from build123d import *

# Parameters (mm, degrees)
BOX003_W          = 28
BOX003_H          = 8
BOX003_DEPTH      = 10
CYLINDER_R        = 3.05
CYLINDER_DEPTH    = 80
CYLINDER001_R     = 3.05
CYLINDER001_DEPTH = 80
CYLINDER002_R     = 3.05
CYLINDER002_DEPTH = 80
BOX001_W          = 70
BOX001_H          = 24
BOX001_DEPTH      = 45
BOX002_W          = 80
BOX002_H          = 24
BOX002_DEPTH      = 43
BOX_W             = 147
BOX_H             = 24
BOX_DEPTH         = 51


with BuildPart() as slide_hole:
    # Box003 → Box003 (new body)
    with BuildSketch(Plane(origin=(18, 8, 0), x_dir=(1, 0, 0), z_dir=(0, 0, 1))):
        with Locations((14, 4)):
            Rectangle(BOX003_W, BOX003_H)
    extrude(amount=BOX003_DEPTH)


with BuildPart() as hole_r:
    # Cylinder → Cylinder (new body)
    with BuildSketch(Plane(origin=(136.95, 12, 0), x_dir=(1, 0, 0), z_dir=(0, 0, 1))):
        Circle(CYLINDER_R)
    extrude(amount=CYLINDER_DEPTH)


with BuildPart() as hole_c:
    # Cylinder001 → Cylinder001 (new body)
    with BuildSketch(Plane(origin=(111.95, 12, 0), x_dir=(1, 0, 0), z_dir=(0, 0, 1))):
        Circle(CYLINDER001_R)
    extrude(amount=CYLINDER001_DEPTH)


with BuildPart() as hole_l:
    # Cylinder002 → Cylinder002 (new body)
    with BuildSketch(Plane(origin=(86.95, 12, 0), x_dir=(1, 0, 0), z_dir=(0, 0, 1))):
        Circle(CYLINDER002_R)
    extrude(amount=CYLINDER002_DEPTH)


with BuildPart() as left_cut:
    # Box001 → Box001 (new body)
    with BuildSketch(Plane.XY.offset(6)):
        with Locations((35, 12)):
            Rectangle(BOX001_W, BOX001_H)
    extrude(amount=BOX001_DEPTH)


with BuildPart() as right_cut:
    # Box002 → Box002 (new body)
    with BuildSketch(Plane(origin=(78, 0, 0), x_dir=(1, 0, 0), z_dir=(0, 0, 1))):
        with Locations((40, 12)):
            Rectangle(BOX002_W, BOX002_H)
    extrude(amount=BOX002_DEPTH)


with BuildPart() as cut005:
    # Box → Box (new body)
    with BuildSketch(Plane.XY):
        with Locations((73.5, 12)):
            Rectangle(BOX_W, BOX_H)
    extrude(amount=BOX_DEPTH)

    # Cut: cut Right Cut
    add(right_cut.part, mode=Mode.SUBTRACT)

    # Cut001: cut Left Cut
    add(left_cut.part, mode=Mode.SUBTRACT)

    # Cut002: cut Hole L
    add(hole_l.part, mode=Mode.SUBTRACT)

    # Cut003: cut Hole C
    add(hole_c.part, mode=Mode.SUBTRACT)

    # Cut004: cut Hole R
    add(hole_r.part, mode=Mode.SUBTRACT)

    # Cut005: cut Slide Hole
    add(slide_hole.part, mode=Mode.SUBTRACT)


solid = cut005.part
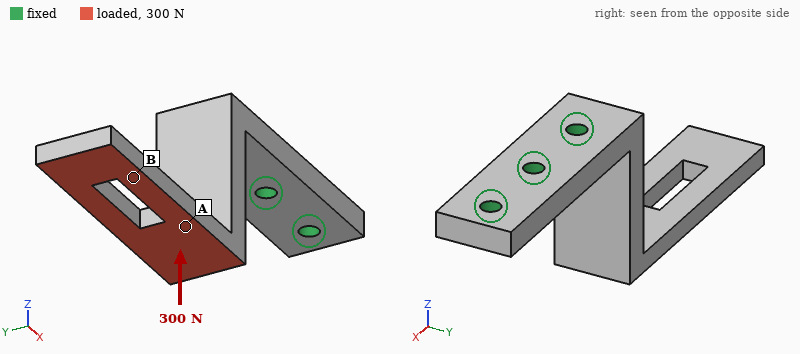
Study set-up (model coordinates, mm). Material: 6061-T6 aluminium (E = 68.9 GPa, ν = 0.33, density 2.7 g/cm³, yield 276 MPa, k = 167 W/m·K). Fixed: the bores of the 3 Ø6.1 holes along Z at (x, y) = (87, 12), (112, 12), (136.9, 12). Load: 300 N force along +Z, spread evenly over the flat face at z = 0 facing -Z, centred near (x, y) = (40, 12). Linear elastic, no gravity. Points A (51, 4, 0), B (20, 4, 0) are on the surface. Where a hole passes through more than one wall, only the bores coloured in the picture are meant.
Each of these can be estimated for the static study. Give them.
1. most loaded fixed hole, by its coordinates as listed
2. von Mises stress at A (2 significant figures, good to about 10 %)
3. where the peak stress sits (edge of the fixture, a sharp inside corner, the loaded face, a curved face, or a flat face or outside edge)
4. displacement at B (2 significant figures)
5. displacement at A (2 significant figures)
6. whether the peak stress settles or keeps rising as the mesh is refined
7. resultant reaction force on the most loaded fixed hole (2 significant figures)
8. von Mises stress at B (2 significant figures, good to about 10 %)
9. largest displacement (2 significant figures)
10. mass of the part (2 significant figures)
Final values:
(87, 12)
39 MPa
edge of the fixture
0.79 mm
0.36 mm
keeps rising
420 N
8.6 MPa
1.1 mm
84 g
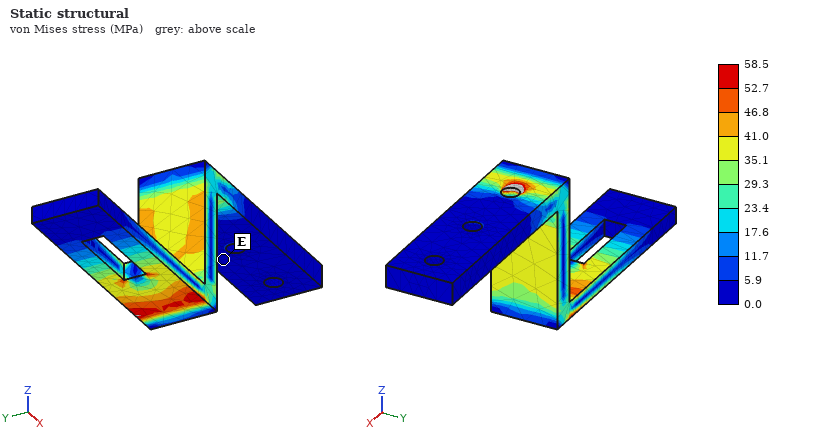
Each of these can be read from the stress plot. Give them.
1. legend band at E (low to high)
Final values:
0.0 to 5.9 MPa
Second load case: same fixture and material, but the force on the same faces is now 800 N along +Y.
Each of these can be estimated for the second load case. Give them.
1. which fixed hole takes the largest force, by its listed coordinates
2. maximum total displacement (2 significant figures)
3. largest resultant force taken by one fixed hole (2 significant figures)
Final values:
(87, 12)
1.2 mm
1.7 kN
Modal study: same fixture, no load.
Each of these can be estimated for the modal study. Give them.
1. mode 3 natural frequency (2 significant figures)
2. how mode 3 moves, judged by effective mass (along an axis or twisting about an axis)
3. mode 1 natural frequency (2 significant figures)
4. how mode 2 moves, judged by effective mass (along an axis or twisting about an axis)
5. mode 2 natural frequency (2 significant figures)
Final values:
1500 Hz
along X
580 Hz
along Y
940 Hz
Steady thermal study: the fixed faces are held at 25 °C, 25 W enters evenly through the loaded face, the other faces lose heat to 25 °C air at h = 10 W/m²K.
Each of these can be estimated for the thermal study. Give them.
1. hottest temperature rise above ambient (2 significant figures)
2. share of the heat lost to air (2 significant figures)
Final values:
74 K
9.9 %
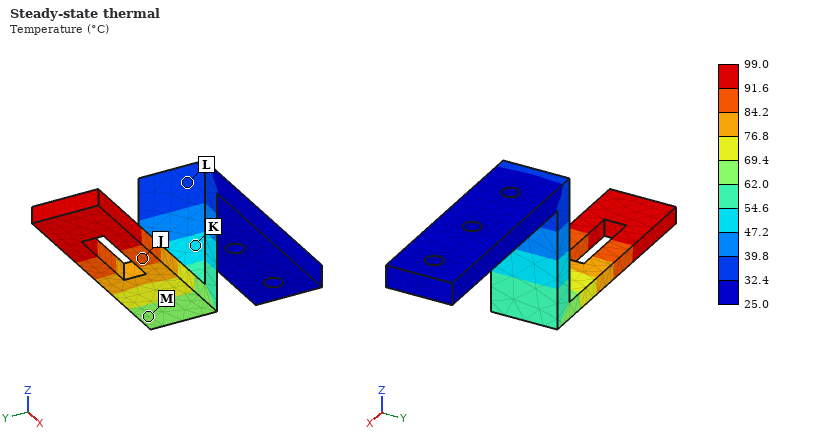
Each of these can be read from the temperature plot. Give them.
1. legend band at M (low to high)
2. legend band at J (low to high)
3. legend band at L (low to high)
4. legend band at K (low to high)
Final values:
62.0 to 69.4 °C
84.2 to 91.6 °C
32.4 to 39.8 °C
47.2 to 54.6 °C
